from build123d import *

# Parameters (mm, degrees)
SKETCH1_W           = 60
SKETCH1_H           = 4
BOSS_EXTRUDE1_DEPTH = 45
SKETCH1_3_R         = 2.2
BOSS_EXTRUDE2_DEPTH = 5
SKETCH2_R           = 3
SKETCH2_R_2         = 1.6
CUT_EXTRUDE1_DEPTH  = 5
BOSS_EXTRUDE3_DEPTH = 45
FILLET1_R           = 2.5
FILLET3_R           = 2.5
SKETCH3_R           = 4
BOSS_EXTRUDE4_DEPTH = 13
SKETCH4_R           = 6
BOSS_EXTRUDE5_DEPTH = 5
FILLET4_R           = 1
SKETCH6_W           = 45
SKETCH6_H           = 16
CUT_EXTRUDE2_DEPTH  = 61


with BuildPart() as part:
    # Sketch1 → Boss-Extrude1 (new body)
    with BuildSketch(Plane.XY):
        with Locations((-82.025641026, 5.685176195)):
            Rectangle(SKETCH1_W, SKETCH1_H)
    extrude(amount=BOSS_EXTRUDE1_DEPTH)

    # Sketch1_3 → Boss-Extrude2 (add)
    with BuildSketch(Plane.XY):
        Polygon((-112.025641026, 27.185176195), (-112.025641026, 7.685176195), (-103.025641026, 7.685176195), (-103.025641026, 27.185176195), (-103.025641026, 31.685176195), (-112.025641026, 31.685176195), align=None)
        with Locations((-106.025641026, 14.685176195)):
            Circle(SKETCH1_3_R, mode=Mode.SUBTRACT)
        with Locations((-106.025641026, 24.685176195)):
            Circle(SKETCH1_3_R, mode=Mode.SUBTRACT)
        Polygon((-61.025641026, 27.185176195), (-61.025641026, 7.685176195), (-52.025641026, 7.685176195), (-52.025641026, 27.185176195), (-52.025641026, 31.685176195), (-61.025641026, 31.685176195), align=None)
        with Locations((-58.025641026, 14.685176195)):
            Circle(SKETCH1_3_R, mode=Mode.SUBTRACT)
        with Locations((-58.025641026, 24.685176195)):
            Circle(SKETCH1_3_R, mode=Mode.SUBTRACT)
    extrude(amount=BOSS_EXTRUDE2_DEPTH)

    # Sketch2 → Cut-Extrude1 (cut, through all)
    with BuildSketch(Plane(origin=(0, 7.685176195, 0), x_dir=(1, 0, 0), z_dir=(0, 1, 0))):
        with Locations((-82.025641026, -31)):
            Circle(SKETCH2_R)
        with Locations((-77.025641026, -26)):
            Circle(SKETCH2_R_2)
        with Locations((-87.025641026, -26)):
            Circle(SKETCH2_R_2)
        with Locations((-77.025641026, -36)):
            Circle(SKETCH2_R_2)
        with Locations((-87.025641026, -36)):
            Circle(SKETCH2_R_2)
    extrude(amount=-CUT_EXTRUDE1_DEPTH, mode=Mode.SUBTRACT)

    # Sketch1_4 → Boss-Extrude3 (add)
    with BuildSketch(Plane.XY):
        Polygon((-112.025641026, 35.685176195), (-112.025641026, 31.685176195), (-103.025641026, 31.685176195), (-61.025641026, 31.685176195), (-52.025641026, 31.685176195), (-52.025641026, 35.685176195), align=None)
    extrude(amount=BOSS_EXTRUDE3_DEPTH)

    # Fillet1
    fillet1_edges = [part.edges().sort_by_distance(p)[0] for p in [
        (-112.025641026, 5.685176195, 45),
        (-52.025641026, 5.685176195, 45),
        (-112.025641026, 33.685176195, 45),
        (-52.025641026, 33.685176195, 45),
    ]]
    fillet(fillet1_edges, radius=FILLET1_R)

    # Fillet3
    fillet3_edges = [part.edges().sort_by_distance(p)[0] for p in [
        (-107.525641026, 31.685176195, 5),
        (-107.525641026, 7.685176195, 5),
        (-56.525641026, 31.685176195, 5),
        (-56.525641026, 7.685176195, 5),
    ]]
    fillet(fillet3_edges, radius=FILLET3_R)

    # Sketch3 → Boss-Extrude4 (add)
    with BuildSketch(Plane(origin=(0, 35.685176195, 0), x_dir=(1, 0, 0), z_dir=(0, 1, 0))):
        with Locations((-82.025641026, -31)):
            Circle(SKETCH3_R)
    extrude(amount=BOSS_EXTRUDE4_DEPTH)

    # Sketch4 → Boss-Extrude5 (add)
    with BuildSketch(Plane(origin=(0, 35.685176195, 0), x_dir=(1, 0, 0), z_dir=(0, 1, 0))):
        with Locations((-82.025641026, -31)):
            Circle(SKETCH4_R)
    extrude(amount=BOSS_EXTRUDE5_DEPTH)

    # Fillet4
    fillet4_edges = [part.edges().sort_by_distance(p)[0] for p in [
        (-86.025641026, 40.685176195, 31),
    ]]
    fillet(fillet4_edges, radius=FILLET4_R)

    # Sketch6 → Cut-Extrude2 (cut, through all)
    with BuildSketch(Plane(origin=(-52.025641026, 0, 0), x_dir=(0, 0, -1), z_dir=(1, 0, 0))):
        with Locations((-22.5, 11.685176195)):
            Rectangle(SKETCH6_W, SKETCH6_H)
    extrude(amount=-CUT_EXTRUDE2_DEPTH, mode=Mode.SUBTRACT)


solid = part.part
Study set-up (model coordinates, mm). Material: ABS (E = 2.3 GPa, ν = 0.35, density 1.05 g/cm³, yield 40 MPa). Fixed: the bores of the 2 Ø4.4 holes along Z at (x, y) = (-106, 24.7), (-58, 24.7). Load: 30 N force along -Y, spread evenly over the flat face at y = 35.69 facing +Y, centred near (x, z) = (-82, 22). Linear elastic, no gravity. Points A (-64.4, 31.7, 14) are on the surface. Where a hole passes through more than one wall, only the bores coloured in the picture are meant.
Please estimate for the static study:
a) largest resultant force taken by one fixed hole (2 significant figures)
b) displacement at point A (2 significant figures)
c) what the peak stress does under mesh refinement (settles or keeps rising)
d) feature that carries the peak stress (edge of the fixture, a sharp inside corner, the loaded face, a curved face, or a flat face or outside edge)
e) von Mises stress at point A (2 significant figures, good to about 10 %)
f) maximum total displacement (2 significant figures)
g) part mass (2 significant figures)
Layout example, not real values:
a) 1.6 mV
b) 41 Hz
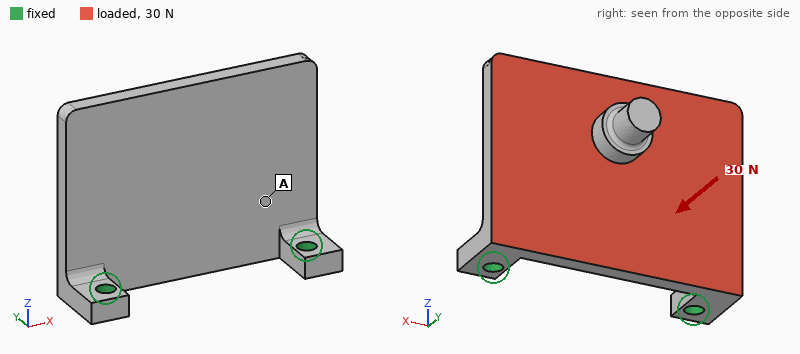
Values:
a) 16 N
b) 0.17 mm
c) keeps rising
d) a sharp inside corner
e) 2.0 MPa
f) 0.85 mm
g) 13 g
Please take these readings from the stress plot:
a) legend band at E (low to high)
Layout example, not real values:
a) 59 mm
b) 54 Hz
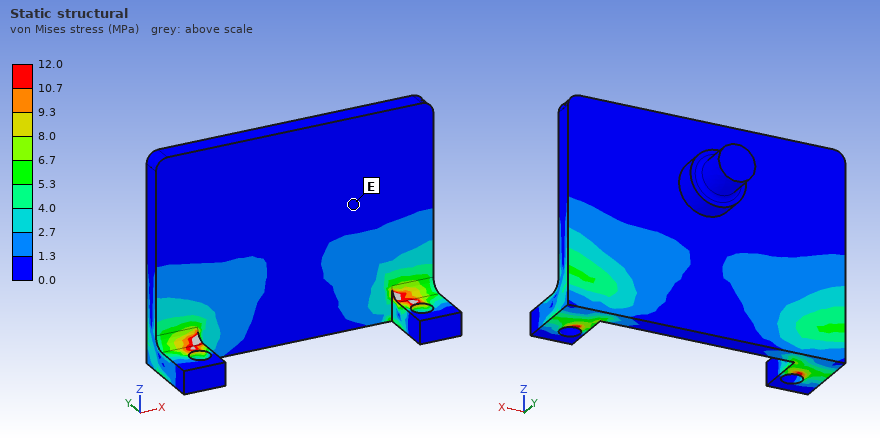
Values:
a) 0.0 to 1.3 MPa
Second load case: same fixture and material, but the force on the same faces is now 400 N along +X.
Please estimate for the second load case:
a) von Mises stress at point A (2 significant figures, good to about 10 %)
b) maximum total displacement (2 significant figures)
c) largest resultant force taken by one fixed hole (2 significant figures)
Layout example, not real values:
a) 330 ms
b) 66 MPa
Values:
a) 4.8 MPa
b) 0.33 mm
c) 250 N
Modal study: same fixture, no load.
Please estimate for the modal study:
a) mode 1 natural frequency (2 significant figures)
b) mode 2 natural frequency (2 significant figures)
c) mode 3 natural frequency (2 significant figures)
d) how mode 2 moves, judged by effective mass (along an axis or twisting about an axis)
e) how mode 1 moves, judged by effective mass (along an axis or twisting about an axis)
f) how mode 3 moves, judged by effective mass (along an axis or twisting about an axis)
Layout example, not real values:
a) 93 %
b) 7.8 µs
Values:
a) 320 Hz
b) 930 Hz
c) 1800 Hz
d) twisting about Z
e) along Y
f) along X
